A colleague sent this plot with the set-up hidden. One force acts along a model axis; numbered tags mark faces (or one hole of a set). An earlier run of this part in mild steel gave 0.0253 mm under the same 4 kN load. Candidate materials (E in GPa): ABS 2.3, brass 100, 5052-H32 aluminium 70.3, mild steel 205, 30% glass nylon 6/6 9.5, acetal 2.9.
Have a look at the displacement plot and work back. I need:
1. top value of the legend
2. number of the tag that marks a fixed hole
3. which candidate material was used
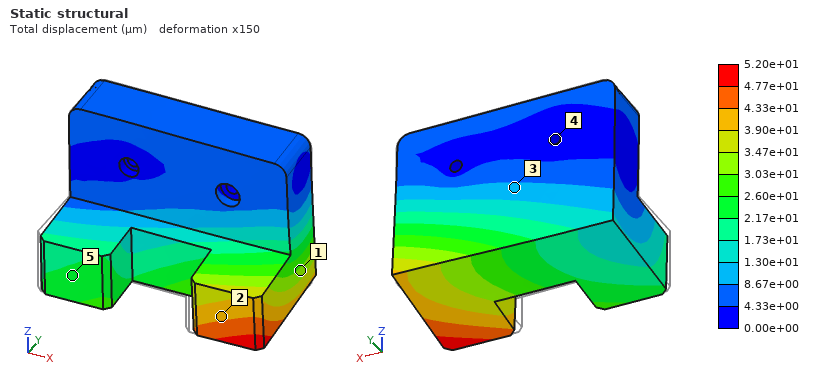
5.20e+01 µm
4
brass
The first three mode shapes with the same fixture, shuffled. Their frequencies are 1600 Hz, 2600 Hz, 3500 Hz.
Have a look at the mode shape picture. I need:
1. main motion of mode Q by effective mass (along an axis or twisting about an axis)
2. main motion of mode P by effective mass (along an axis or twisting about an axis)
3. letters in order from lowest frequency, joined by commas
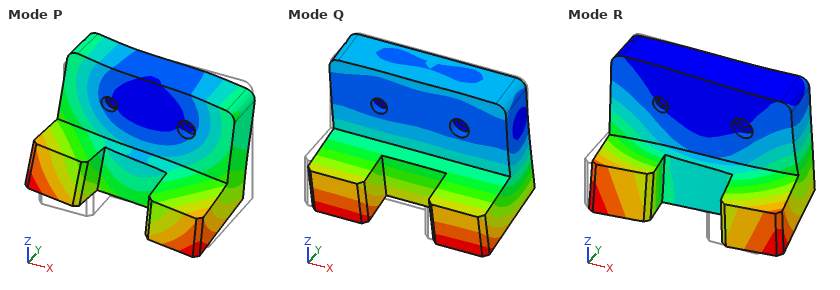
along Y
along X
Q, R, P
